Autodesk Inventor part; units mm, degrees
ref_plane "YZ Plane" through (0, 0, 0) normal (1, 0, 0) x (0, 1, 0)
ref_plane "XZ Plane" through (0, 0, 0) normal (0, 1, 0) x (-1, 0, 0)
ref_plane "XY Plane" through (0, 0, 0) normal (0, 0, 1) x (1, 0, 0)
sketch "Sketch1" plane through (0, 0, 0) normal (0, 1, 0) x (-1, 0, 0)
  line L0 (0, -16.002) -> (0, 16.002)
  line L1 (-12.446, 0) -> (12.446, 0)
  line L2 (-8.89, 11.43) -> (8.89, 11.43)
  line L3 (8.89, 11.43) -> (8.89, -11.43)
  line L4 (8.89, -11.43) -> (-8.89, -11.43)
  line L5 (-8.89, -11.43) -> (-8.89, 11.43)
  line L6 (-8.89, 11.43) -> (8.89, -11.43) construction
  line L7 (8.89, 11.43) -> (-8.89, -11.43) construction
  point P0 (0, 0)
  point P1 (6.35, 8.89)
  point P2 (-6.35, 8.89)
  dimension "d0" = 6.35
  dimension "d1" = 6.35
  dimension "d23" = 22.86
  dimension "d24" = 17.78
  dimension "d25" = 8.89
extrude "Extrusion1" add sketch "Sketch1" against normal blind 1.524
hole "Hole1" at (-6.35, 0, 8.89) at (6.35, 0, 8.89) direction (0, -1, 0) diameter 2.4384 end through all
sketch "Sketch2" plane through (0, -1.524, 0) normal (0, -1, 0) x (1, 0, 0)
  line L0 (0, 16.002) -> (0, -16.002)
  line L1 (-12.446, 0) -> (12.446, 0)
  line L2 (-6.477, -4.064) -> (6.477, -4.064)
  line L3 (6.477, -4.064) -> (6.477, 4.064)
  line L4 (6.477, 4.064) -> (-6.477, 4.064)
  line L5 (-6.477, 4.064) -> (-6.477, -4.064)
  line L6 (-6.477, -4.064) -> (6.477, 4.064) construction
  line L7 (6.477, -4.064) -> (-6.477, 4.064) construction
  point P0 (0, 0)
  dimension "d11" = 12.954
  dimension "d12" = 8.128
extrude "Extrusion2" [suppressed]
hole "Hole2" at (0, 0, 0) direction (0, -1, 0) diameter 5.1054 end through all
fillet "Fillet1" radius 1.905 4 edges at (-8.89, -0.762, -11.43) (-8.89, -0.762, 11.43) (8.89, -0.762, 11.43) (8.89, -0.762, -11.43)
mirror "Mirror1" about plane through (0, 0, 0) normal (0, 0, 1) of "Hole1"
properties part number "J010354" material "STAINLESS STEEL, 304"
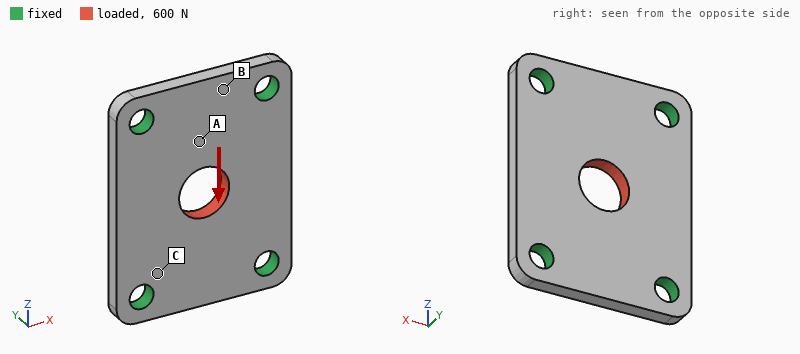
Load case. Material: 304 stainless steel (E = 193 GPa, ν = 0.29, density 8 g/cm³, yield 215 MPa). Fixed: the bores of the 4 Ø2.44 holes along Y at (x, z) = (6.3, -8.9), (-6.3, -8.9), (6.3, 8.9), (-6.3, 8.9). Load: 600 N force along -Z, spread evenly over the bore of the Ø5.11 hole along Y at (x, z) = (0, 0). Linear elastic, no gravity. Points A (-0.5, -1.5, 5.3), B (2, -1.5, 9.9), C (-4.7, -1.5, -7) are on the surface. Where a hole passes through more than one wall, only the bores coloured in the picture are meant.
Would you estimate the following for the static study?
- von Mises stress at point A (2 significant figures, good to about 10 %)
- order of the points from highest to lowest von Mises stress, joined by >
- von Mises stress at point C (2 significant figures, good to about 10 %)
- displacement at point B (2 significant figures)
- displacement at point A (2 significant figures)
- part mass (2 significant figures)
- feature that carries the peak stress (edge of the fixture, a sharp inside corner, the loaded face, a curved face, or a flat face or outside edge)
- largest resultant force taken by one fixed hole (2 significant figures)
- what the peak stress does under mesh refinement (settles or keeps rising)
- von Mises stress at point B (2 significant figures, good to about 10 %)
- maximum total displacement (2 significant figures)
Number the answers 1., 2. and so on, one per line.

1. 14 MPa
2. C > A > B
3. 23 MPa
4. 0.44 µm
5. 0.67 µm
6. 4.4 g
7. edge of the fixture
8. 160 N
9. keeps rising
10. 6.4 MPa
11. 0.96 µm
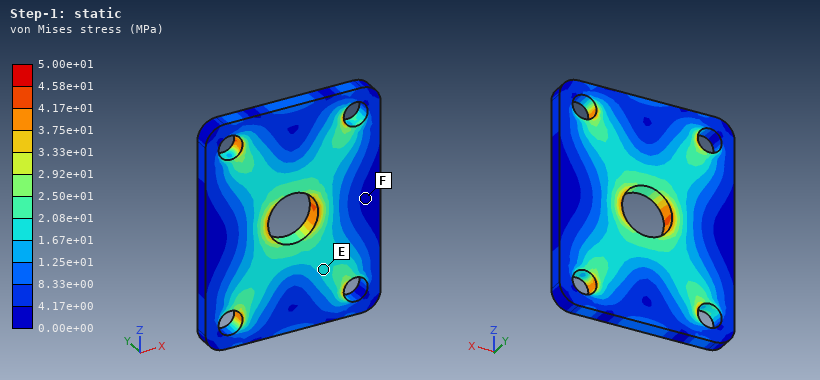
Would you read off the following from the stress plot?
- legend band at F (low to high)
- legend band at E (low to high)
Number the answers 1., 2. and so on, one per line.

1. 0.00e+00 to 4.17e+00 MPa
2. 1.67e+01 to 2.08e+01 MPa
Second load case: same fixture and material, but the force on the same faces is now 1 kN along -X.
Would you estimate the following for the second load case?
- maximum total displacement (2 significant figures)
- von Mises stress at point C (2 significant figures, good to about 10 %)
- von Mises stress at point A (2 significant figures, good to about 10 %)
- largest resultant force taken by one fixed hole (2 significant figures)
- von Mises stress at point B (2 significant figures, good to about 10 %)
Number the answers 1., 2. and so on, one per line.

1. 2.6 µm
2. 45 MPa
3. 39 MPa
4. 290 N
5. 8.6 MPa
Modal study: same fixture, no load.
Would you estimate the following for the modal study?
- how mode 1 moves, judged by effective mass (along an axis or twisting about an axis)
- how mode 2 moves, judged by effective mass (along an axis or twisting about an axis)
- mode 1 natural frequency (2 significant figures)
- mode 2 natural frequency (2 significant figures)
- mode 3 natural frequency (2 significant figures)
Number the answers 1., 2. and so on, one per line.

1. along Y
2. twisting about Z
3. 25 kHz
4. 32 kHz
5. 42 kHz
